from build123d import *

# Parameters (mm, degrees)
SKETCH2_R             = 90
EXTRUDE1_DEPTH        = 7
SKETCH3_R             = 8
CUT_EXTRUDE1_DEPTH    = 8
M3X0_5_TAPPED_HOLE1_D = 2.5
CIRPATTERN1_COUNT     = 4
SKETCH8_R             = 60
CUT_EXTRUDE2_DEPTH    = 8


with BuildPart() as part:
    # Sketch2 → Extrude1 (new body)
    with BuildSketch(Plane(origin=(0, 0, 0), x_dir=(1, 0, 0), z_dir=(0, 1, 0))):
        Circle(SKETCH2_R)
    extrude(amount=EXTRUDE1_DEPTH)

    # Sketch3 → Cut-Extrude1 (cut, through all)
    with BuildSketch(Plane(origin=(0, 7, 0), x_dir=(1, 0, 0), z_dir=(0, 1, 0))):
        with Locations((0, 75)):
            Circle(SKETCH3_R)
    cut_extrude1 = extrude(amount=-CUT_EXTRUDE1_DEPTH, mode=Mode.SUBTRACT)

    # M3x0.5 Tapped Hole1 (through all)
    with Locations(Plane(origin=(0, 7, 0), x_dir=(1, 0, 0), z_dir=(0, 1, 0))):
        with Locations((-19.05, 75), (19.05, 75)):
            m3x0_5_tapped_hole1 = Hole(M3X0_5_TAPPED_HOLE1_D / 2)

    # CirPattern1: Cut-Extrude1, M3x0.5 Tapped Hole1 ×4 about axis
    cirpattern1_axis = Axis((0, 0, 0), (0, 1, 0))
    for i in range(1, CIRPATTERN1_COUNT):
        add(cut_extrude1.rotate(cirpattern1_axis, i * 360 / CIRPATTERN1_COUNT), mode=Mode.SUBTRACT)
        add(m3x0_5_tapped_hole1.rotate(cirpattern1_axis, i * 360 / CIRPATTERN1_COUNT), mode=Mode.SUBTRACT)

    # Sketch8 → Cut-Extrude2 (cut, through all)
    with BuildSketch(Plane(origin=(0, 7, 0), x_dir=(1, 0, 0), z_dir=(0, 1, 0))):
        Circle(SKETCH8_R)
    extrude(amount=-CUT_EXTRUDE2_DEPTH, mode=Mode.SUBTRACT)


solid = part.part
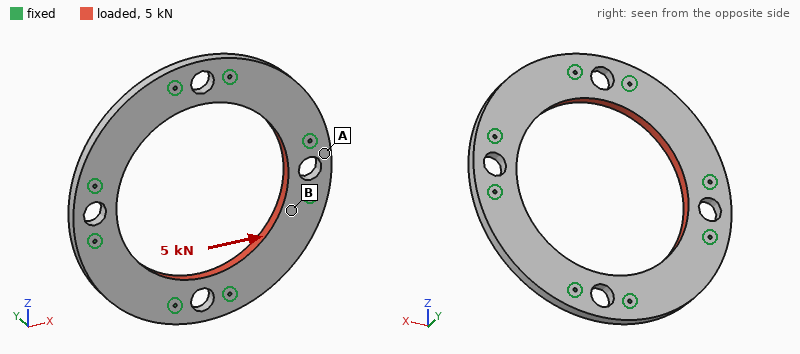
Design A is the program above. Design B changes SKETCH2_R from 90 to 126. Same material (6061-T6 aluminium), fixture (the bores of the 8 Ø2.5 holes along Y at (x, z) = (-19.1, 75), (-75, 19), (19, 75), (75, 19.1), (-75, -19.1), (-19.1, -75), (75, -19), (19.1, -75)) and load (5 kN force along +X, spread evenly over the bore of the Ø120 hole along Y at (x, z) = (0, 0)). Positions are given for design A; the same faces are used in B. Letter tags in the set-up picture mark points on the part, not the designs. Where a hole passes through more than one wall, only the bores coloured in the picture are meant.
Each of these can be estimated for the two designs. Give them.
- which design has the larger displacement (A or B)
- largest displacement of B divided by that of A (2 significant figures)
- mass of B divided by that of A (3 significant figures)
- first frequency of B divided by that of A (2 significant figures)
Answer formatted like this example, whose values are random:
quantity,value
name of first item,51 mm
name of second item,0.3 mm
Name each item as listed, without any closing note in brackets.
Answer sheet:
quantity,value
which design has the larger displacement,A
largest displacement of B divided by that of A,0.58
mass of B divided by that of A,2.84
first frequency of B divided by that of A,0.34
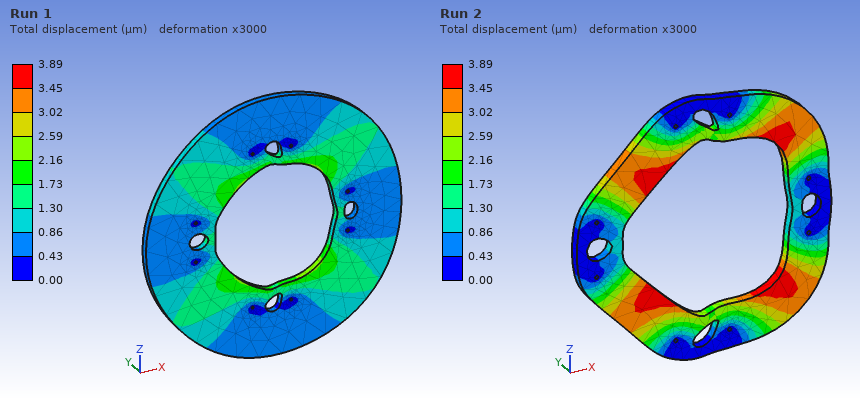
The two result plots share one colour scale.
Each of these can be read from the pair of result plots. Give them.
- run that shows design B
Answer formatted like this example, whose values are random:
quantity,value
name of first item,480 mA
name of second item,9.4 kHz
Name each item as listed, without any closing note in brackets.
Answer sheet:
quantity,value
run that shows design B,Run 1
